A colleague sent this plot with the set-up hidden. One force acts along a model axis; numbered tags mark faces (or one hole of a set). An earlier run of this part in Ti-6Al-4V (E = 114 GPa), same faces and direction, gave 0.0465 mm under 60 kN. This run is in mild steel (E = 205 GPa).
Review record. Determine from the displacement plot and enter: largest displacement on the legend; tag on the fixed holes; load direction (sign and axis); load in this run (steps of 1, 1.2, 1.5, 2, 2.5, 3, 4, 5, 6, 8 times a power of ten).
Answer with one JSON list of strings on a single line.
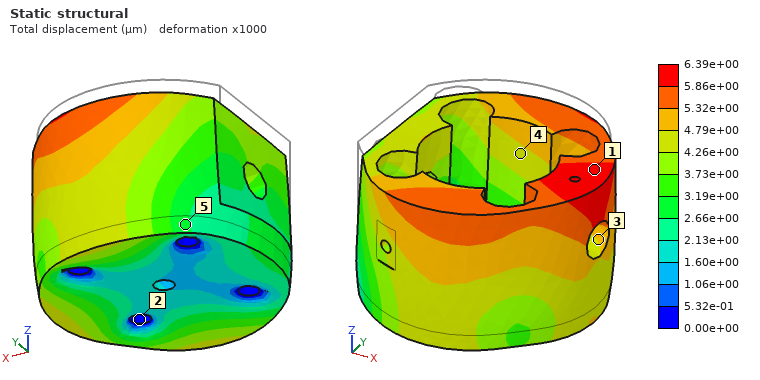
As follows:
["6.39e+00 µm", "2", "-Z", "15 kN"]
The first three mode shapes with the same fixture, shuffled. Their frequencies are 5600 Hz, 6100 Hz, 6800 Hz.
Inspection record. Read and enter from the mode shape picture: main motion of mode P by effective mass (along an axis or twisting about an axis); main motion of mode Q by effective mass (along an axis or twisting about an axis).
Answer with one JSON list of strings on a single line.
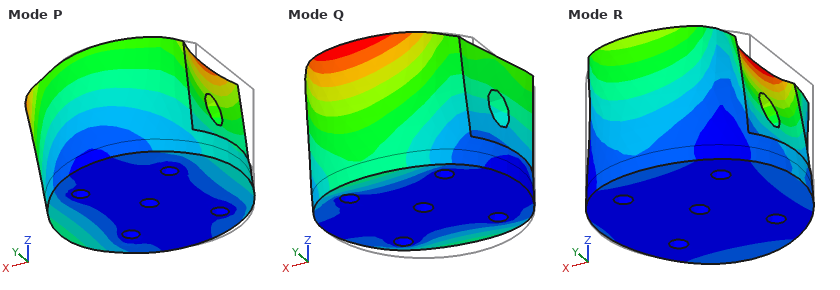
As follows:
["along X", "along Y"]
